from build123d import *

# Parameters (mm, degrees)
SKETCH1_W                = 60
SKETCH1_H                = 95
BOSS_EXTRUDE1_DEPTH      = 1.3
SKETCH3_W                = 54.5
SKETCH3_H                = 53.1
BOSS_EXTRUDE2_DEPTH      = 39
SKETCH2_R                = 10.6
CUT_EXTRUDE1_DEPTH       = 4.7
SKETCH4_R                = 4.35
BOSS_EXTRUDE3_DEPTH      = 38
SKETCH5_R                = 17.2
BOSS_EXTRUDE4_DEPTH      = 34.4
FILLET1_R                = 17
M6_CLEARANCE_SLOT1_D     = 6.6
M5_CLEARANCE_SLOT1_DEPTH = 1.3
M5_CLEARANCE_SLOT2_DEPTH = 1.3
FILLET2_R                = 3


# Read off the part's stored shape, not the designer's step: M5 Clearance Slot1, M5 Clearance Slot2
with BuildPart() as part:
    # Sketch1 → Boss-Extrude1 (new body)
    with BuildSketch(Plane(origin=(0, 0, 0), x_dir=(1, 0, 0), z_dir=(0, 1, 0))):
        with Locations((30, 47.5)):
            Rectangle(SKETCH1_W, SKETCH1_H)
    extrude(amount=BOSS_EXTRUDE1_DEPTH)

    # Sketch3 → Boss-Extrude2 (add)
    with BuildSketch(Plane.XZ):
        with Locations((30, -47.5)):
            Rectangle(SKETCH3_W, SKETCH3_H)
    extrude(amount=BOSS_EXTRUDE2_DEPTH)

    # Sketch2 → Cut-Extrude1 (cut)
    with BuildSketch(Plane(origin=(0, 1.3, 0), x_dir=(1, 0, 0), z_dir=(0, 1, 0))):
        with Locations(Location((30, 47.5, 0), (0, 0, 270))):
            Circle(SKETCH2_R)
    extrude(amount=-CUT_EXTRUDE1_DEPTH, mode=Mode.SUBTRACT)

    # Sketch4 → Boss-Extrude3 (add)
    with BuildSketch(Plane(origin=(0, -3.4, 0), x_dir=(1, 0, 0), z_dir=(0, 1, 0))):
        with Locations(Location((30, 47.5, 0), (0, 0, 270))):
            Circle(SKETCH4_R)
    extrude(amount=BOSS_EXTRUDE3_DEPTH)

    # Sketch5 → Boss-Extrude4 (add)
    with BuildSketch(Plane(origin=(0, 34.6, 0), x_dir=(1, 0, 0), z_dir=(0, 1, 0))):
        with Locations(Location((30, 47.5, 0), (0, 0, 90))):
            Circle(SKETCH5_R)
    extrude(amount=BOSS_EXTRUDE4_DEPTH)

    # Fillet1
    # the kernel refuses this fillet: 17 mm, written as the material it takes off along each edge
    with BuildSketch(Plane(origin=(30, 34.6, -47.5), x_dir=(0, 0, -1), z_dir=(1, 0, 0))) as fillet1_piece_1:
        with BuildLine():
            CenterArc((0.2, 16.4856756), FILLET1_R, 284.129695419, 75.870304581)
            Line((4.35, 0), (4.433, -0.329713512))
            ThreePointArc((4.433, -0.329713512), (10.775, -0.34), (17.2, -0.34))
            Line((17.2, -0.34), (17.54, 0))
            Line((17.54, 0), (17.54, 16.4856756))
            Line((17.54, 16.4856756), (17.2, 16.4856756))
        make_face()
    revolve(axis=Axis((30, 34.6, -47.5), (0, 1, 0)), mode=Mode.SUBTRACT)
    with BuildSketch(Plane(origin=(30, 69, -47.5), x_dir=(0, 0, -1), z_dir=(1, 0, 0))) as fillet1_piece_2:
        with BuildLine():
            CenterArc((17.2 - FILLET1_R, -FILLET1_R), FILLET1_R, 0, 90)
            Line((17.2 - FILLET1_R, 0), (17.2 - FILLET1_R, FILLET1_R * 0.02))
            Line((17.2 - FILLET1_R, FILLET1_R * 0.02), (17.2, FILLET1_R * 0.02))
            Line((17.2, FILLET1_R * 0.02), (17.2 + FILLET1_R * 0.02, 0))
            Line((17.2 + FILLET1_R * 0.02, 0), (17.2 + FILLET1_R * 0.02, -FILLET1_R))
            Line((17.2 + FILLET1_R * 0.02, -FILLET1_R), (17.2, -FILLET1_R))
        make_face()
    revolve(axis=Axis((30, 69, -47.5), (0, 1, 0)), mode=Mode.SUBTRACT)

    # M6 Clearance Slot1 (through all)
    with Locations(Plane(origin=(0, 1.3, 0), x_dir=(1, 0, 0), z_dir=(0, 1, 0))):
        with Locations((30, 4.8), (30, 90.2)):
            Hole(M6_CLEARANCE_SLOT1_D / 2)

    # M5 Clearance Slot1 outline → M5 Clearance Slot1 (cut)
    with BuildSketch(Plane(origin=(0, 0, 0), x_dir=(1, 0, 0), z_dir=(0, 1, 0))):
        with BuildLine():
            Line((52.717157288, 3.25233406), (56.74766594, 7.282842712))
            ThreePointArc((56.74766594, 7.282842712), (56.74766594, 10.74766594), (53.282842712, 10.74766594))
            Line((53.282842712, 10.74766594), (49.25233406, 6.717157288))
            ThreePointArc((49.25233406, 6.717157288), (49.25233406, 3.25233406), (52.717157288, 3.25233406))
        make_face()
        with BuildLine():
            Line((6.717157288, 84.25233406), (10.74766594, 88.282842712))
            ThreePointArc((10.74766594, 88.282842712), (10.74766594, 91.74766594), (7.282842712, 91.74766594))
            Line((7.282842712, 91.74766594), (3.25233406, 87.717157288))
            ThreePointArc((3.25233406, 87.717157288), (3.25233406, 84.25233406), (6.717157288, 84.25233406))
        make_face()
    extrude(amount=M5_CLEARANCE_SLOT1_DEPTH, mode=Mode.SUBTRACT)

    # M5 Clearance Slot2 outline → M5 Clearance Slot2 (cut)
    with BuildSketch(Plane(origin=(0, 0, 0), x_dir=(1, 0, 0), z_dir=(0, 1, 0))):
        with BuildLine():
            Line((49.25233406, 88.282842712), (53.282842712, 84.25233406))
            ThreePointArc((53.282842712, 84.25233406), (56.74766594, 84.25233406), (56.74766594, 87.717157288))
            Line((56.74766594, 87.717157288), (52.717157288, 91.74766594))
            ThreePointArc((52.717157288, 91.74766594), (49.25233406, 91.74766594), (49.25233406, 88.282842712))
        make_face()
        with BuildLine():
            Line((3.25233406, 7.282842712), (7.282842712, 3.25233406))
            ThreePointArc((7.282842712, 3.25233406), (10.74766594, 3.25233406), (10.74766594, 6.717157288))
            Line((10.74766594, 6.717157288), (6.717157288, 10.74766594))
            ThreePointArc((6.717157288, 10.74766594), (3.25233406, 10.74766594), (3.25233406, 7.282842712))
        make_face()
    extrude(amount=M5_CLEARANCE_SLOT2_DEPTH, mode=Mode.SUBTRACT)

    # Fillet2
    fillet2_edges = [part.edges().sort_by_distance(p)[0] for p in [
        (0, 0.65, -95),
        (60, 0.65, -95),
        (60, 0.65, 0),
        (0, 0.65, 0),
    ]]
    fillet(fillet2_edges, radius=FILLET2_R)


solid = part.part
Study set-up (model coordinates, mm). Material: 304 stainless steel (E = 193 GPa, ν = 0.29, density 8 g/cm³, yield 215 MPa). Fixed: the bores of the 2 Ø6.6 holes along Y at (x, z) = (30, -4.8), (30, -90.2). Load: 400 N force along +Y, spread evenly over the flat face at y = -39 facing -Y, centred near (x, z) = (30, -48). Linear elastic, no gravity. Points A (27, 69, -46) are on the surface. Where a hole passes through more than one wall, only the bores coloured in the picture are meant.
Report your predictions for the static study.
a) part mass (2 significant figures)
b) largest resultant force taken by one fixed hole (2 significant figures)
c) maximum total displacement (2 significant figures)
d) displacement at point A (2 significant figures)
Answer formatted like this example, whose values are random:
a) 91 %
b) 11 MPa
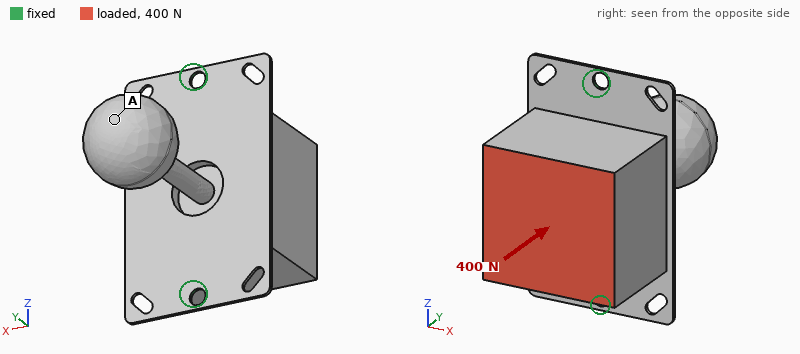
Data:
a) 1.1 kg
b) 230 N
c) 56 µm
d) 54 µm
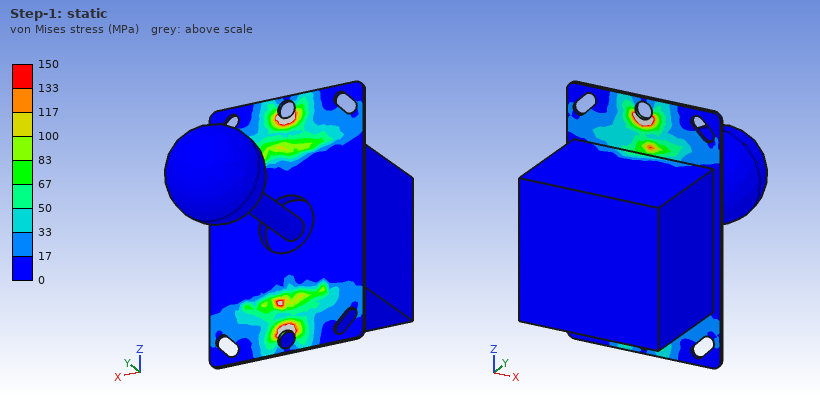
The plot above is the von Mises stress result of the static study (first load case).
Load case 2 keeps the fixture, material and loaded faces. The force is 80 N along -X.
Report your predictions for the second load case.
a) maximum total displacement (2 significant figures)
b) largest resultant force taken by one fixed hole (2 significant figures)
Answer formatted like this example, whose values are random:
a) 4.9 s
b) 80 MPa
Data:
a) 0.46 mm
b) 40 N
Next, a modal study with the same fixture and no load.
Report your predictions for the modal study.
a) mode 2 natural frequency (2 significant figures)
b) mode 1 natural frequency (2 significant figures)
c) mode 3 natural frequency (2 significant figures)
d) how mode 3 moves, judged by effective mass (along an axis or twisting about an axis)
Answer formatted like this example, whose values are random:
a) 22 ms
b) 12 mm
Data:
a) 300 Hz
b) 98 Hz
c) 410 Hz
d) along Y
